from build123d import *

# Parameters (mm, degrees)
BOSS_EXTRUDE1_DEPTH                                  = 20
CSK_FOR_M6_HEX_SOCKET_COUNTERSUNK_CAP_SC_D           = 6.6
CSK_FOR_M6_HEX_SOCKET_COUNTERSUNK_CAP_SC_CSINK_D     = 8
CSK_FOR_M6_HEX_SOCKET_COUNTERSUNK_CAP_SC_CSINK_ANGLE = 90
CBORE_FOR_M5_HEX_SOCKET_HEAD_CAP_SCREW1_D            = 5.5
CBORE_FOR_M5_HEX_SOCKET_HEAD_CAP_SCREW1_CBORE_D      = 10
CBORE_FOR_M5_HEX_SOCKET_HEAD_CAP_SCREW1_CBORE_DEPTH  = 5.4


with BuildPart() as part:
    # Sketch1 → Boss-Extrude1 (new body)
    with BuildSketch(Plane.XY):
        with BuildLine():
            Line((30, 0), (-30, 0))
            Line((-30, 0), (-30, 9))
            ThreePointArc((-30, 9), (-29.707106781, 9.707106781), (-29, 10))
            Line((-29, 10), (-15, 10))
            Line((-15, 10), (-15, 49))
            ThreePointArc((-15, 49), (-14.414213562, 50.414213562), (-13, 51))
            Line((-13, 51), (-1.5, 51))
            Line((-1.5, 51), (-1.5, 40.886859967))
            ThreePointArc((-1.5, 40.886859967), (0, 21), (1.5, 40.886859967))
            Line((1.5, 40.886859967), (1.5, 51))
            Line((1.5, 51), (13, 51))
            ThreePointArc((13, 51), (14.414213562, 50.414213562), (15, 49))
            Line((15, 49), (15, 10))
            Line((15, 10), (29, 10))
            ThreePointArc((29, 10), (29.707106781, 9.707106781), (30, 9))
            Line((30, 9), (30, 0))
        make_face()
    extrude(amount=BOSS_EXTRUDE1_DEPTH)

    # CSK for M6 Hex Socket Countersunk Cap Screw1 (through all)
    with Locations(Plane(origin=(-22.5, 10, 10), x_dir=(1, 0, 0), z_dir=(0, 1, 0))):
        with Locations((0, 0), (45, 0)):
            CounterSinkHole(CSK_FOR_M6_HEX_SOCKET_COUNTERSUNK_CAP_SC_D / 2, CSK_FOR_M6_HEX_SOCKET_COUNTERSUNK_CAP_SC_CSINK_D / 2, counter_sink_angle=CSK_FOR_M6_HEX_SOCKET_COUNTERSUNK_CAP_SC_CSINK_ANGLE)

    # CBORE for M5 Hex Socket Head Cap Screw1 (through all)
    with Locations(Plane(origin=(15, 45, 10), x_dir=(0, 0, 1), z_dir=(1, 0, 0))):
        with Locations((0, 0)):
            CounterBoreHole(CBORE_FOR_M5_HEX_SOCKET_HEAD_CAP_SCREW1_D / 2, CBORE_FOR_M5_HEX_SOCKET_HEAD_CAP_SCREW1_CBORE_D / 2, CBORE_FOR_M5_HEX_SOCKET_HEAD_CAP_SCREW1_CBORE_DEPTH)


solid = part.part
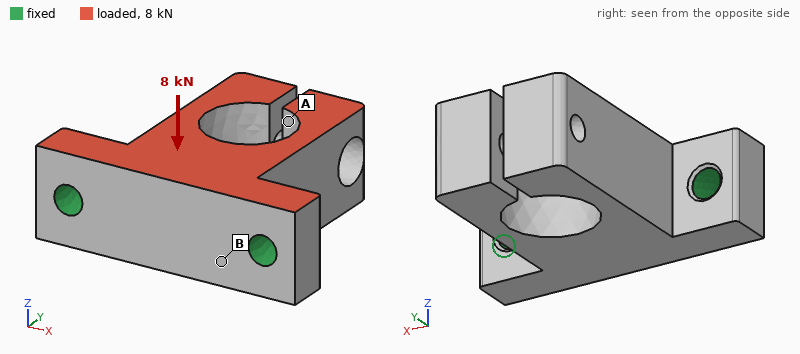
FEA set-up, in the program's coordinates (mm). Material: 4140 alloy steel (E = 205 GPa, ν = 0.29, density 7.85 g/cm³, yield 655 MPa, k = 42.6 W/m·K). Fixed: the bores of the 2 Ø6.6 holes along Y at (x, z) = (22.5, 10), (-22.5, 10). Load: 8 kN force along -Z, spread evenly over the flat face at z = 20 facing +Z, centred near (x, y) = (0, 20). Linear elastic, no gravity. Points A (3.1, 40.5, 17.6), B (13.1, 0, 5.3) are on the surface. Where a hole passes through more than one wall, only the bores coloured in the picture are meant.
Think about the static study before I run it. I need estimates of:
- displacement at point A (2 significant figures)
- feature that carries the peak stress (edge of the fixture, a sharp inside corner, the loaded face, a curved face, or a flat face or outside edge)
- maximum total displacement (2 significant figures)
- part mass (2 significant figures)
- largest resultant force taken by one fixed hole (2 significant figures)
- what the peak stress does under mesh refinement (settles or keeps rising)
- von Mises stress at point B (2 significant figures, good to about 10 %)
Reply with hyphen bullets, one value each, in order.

- 0.076 mm
- edge of the fixture
- 0.10 mm
- 220 g
- 4.0 kN
- keeps rising
- 66 MPa
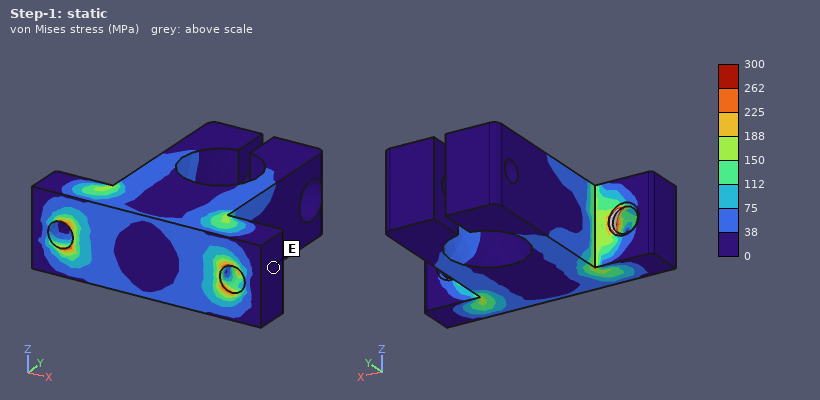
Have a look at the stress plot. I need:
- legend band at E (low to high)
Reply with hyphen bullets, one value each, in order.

- 0 to 38 MPa
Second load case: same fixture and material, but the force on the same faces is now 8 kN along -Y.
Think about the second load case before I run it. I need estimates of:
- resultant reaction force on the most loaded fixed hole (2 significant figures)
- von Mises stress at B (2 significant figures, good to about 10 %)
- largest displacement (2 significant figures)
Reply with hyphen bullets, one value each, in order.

- 4.2 kN
- 49 MPa
- 61 µm
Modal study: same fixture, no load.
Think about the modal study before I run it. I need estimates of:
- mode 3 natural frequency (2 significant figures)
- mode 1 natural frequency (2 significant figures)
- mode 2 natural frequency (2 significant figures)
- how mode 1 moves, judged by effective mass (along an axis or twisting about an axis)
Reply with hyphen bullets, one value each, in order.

- 3800 Hz
- 3600 Hz
- 3700 Hz
- along X
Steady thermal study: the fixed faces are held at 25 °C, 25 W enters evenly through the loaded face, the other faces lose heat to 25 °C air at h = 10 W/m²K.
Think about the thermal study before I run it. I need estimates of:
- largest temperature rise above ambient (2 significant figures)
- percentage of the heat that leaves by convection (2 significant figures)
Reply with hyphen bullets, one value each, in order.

- 36 K
- 5.9 %
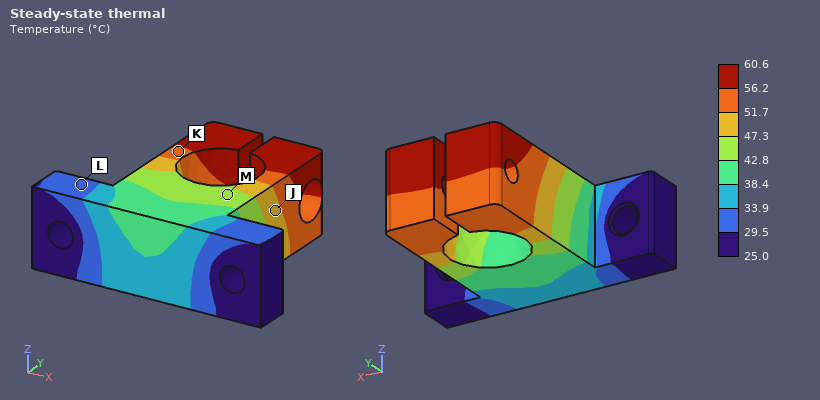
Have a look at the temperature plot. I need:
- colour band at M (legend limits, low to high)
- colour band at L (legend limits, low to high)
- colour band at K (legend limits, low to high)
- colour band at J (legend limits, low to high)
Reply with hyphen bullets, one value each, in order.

- 42.8 to 47.3 °C
- 29.5 to 33.9 °C
- 51.7 to 56.2 °C
- 47.3 to 51.7 °C
